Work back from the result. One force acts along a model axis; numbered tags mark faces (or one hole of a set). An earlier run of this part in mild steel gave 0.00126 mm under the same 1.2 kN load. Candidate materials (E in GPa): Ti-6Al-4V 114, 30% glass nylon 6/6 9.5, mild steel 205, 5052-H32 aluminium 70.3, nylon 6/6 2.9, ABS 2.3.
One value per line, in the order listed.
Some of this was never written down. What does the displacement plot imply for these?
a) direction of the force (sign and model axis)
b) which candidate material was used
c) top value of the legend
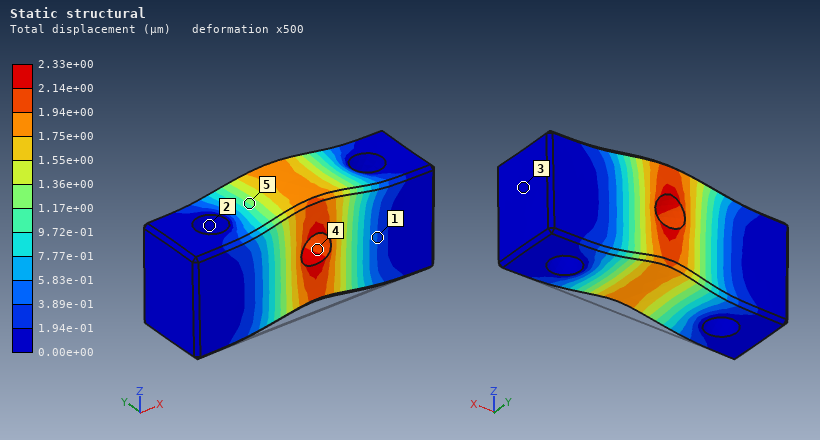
+Z
Ti-6Al-4V
2.33e+00 µm
